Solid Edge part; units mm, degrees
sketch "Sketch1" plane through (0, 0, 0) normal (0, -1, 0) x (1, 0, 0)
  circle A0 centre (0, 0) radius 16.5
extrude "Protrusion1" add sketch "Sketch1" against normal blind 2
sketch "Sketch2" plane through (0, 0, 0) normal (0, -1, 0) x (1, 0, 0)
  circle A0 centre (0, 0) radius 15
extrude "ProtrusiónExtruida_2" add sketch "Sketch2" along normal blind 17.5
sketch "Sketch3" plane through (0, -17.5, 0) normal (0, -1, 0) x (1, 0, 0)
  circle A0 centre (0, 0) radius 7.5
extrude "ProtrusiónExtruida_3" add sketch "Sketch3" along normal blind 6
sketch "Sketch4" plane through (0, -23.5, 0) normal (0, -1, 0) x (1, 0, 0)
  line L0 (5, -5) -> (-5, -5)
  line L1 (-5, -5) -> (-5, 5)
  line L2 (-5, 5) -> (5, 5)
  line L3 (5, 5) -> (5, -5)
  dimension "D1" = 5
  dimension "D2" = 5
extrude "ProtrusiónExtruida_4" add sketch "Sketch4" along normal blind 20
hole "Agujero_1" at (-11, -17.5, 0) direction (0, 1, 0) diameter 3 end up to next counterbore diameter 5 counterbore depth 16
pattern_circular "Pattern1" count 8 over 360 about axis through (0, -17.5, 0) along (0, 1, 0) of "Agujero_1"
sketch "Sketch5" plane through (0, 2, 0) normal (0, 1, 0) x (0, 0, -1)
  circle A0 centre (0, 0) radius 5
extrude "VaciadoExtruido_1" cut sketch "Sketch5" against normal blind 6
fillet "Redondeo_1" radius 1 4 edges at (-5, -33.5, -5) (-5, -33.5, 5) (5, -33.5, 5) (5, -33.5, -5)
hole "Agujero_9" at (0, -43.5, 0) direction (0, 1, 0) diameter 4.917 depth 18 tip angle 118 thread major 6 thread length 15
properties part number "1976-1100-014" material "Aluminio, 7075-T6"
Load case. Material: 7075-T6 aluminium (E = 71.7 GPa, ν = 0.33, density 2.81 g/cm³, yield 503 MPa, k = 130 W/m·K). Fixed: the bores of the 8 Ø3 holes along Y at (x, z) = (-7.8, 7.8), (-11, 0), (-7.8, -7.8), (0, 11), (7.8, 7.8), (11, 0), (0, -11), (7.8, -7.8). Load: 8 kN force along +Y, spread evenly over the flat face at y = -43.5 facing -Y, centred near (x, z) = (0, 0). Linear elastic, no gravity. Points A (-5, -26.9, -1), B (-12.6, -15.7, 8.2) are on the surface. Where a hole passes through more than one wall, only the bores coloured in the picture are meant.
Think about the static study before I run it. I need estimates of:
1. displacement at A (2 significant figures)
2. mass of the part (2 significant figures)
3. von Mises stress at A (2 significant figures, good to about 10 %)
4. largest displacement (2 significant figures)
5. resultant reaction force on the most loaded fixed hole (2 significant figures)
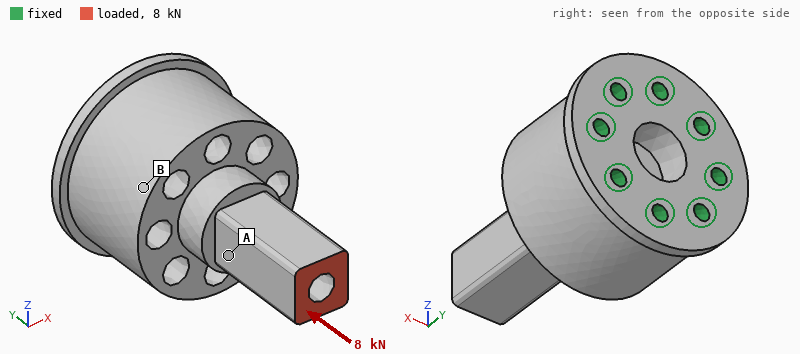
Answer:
17 µm
38 g
93 MPa
40 µm
1.1 kN
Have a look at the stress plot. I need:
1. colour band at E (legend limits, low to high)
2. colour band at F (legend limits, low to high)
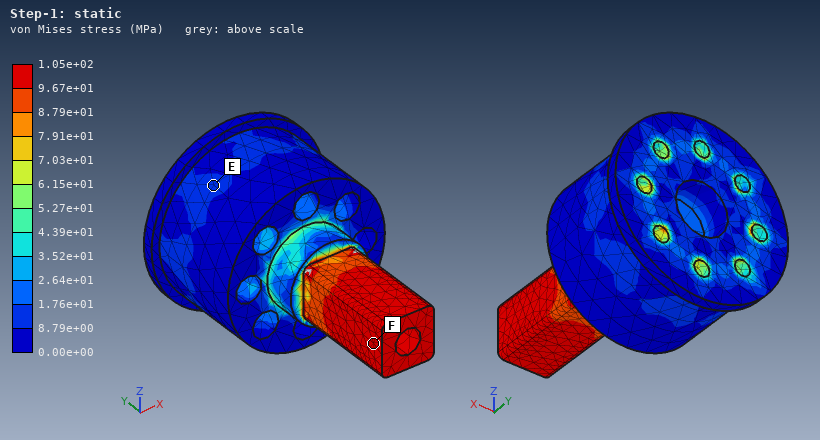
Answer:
8.79e+00 to 1.76e+01 MPa
9.67e+01 to 1.05e+02 MPa
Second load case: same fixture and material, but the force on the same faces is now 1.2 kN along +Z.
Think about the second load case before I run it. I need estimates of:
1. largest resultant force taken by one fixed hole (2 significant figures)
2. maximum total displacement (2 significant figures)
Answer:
1.1 kN
0.15 mm
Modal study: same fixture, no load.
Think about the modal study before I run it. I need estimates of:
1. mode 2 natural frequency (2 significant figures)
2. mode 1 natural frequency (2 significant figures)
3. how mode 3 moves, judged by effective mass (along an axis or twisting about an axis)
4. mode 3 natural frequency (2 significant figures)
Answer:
11 kHz
11 kHz
along X
24 kHz
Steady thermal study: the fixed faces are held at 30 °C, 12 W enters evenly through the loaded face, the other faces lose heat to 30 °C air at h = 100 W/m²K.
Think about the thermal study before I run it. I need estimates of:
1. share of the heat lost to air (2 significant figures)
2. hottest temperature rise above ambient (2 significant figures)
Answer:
22 %
28 K
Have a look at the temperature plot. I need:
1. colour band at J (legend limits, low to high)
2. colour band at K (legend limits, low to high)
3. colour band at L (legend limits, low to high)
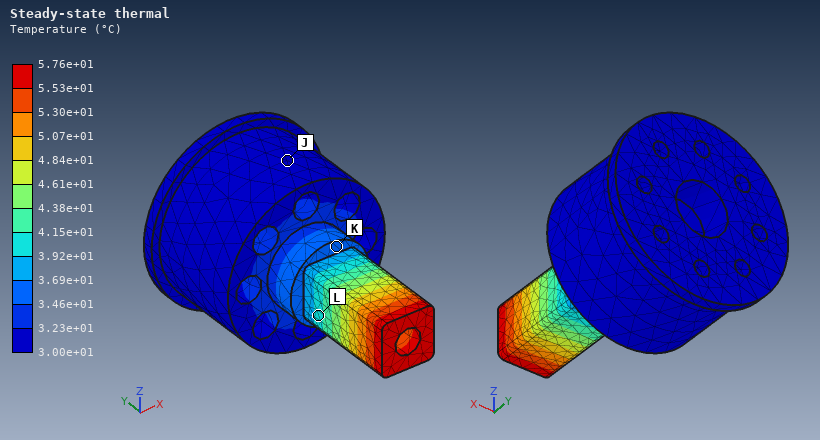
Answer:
3.00e+01 to 3.23e+01 °C
3.46e+01 to 3.69e+01 °C
3.92e+01 to 4.15e+01 °C
